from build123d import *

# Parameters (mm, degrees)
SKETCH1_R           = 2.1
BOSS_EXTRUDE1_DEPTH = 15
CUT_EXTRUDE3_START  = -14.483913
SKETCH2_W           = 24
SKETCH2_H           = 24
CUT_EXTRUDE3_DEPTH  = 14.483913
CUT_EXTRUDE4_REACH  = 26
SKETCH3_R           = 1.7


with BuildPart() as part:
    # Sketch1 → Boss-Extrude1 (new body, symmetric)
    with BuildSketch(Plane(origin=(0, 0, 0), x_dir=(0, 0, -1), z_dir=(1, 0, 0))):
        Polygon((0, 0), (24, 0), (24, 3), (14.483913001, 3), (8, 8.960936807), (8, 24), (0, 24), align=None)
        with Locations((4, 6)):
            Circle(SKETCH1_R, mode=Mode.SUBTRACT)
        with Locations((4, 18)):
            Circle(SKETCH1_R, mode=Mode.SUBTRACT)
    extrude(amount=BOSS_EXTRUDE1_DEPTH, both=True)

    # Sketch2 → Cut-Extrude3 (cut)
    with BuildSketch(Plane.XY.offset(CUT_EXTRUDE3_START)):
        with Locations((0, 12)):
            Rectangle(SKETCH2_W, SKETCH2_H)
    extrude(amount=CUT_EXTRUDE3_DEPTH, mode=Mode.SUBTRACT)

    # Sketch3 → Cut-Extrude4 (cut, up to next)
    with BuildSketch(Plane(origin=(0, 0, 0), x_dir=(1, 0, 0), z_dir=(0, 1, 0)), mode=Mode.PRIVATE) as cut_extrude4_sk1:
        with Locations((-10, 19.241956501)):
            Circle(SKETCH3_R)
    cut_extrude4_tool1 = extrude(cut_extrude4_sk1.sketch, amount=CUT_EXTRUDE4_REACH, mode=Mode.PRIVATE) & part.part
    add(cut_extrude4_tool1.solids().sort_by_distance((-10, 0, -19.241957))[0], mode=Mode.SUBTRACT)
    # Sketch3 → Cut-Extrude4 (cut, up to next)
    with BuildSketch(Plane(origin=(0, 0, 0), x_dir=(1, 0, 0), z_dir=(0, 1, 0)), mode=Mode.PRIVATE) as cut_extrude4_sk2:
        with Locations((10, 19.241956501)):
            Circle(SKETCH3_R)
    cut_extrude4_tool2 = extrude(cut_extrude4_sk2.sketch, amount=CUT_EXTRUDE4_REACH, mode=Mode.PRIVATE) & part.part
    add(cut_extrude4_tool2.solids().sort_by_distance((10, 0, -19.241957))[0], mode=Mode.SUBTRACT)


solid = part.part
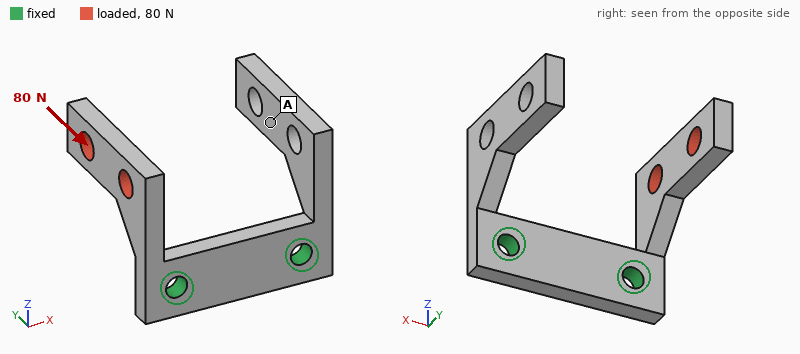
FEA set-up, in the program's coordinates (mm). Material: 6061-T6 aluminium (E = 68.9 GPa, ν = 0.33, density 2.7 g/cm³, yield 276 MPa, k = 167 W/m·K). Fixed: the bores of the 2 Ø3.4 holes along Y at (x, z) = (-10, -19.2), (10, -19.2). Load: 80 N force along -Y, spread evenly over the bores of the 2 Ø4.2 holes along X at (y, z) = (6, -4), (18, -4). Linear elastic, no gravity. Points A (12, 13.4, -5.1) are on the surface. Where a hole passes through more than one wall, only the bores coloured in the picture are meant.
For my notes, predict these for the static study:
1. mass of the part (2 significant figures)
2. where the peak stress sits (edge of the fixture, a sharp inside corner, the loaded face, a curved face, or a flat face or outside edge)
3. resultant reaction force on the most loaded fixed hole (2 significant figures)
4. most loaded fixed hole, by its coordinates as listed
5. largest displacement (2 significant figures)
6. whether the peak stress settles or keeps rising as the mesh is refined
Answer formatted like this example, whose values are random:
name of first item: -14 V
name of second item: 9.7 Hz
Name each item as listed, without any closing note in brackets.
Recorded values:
mass of the part: 5.5 g
where the peak stress sits: a sharp inside corner
resultant reaction force on the most loaded fixed hole: 84 N
most loaded fixed hole, by its coordinates as listed: (-10, -19.2)
largest displacement: 0.26 mm
whether the peak stress settles or keeps rising as the mesh is refined: keeps rising
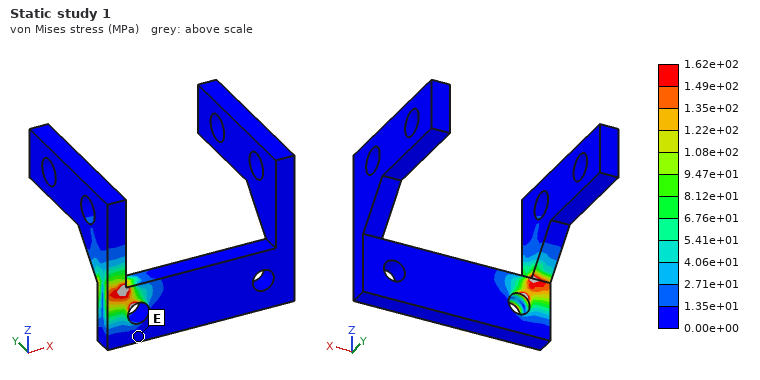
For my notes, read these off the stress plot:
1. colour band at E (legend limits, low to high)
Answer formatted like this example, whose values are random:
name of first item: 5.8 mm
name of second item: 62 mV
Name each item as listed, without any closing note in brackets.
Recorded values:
colour band at E: 0.00e+00 to 1.35e+01 MPa
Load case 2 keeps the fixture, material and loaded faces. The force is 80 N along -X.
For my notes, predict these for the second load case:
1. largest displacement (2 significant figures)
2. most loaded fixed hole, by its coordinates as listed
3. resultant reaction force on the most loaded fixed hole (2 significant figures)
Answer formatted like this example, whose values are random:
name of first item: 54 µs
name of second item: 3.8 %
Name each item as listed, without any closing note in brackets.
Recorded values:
largest displacement: 0.47 mm
most loaded fixed hole, by its coordinates as listed: (-10, -19.2)
resultant reaction force on the most loaded fixed hole: 67 N
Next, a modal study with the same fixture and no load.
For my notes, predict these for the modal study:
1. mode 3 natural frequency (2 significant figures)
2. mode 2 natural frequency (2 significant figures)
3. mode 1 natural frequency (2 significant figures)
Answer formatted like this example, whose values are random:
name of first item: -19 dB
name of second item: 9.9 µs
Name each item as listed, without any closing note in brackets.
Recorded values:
mode 3 natural frequency: 2400 Hz
mode 2 natural frequency: 2200 Hz
mode 1 natural frequency: 2200 Hz
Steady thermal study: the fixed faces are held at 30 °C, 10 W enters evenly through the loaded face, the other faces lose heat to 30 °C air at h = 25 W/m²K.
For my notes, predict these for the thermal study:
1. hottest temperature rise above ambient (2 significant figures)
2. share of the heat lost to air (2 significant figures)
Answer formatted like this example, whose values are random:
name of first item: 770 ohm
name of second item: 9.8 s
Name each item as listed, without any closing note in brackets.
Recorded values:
hottest temperature rise above ambient: 71 K
share of the heat lost to air: 8.7 %
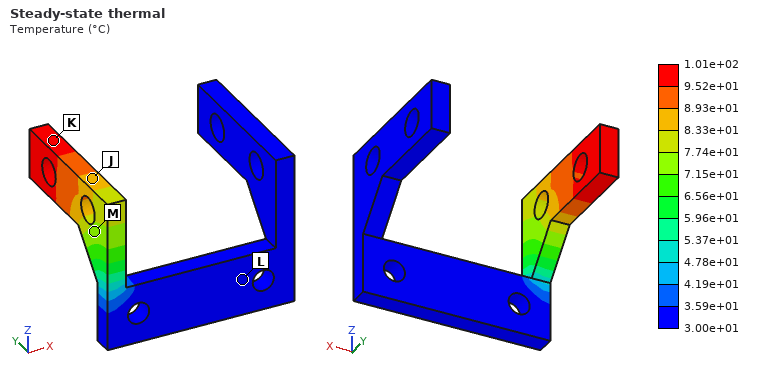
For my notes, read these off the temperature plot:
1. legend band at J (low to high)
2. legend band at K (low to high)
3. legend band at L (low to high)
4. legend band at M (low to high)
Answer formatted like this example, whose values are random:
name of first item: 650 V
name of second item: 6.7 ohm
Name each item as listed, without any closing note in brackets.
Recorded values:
legend band at J: 8.33e+01 to 8.93e+01 °C
legend band at K: 9.52e+01 to 1.01e+02 °C
legend band at L: 3.00e+01 to 3.59e+01 °C
legend band at M: 7.15e+01 to 7.74e+01 °C
